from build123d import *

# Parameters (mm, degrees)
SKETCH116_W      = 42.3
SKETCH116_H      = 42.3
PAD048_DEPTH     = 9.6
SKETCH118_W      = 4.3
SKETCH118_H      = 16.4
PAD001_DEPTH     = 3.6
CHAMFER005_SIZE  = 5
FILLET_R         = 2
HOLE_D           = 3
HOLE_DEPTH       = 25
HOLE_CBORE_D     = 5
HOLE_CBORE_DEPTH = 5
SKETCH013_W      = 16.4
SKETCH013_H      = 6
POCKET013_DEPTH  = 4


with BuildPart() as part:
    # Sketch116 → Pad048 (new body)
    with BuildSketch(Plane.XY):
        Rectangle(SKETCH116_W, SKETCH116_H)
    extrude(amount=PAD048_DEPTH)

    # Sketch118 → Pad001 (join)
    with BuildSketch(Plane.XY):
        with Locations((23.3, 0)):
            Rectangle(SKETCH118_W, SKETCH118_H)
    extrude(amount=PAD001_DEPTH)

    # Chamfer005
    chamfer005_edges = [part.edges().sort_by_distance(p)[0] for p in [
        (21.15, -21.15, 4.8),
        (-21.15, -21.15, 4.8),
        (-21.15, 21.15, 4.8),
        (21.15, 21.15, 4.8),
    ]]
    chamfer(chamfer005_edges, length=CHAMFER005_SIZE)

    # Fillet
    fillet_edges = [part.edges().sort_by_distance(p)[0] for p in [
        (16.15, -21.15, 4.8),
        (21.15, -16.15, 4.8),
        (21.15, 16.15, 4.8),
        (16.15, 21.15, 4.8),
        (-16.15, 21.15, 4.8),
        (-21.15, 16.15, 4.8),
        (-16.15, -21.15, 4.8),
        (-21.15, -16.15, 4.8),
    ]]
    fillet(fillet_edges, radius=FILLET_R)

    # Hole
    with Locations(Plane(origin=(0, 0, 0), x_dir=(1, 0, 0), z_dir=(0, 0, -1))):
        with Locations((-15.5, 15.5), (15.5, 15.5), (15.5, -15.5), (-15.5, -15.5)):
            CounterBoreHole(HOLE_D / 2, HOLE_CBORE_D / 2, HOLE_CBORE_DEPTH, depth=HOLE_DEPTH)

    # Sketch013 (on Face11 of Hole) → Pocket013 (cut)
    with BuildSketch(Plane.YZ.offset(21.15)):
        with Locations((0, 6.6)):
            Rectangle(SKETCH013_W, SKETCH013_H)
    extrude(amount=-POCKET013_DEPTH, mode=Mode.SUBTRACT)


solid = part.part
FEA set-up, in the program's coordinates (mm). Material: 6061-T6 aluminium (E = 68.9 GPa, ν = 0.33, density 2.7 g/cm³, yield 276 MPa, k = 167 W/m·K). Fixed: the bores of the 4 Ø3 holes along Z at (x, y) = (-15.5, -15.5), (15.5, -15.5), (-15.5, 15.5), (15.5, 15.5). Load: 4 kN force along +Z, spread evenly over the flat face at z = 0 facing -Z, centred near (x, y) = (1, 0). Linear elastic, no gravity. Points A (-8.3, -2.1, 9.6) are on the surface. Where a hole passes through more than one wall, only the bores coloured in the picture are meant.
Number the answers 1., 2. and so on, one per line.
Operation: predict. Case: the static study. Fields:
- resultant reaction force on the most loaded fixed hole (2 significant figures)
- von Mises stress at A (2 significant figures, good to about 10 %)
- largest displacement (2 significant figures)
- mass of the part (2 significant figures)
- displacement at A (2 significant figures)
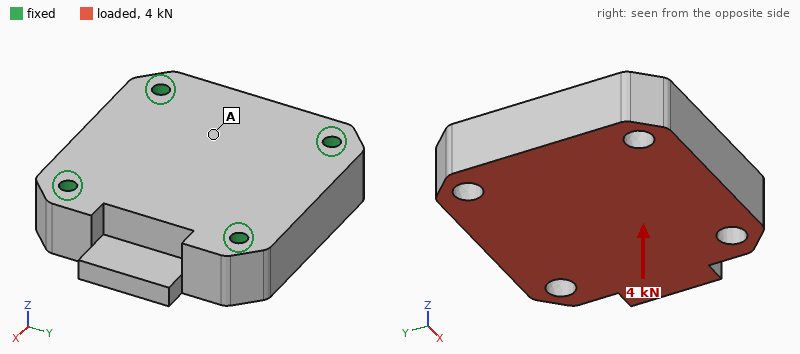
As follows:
1. 1.2 kN
2. 8.1 MPa
3. 12 µm
4. 43 g
5. 6.4 µm
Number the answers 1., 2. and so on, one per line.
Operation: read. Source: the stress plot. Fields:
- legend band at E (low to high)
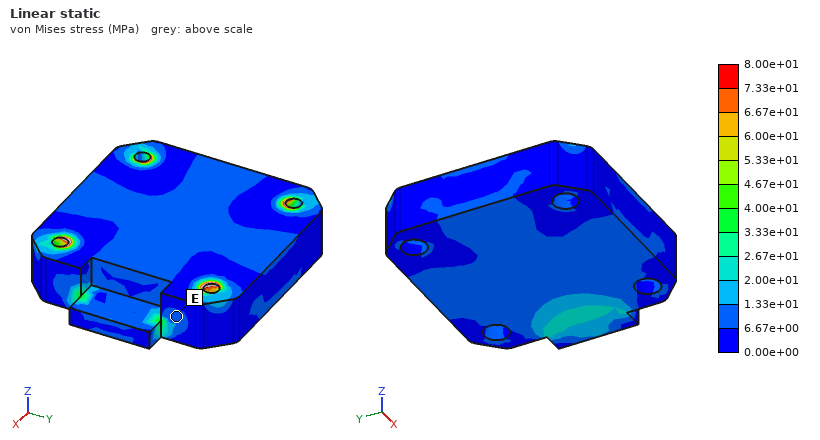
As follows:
1. 6.67e+00 to 1.33e+01 MPa
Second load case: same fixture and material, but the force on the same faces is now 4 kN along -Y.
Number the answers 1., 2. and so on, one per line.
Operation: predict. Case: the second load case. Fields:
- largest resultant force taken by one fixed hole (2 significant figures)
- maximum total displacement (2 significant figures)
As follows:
1. 1.1 kN
2. 6.0 µm
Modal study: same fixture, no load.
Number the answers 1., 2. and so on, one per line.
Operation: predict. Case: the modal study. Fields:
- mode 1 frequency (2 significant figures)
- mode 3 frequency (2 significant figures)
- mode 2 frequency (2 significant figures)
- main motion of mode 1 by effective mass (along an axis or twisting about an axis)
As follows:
1. 20 kHz
2. 28 kHz
3. 26 kHz
4. along Z
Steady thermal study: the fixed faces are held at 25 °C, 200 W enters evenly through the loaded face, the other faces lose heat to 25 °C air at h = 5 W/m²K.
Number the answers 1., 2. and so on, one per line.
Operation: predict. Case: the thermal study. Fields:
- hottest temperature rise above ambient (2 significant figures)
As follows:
1. 31 K
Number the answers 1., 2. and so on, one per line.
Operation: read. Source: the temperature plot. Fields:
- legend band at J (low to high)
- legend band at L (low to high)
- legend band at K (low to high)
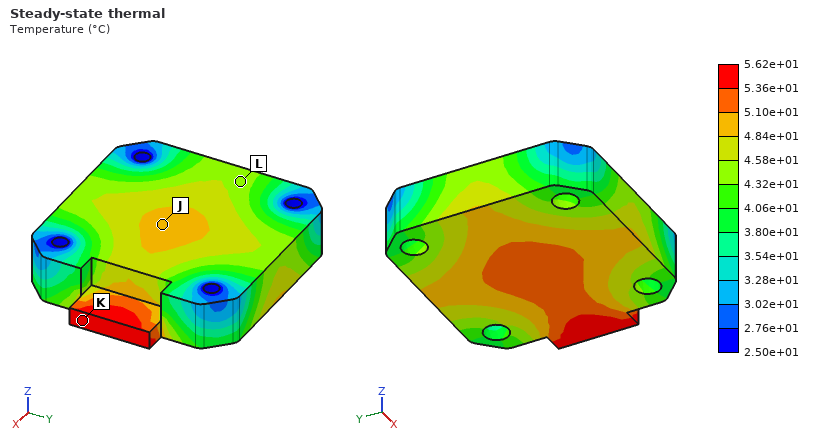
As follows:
1. 4.84e+01 to 5.10e+01 °C
2. 4.32e+01 to 4.58e+01 °C
3. 5.36e+01 to 5.62e+01 °C
